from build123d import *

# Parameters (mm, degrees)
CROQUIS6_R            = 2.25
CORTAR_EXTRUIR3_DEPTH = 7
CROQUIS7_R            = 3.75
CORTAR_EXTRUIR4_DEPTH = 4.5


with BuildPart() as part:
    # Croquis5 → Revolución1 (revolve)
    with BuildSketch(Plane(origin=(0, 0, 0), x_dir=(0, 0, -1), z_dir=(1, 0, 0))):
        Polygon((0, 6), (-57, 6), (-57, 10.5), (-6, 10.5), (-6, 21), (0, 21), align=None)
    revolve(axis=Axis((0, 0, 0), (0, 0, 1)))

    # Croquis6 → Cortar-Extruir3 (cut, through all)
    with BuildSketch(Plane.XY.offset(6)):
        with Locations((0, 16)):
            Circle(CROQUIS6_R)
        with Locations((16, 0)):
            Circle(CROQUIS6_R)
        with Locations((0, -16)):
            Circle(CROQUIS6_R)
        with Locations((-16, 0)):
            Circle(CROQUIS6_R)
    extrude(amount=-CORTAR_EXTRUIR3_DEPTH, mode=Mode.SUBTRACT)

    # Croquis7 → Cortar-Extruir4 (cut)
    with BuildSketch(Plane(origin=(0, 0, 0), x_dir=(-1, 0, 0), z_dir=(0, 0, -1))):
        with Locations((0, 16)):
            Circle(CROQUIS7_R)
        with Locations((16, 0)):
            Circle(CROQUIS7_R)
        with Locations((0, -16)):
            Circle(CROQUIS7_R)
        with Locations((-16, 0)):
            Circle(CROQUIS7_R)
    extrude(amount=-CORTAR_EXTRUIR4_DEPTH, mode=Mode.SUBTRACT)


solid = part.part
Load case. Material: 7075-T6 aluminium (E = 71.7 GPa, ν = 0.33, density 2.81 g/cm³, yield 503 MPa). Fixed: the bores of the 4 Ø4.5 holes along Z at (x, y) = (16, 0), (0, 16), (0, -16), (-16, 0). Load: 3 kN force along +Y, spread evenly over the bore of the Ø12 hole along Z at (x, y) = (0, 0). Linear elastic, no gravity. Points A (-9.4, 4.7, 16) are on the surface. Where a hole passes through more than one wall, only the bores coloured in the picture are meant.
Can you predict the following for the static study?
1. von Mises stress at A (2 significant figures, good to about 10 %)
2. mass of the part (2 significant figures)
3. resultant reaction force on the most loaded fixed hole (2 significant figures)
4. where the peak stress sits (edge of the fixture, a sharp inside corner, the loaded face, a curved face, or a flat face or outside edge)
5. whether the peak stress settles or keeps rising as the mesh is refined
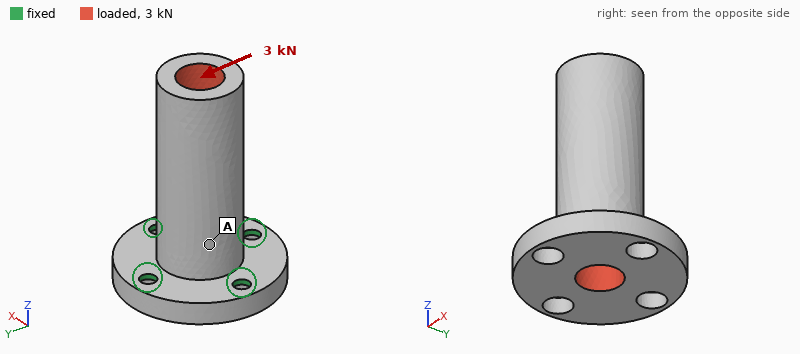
30 MPa
52 g
2.2 kN
edge of the fixture
keeps rising
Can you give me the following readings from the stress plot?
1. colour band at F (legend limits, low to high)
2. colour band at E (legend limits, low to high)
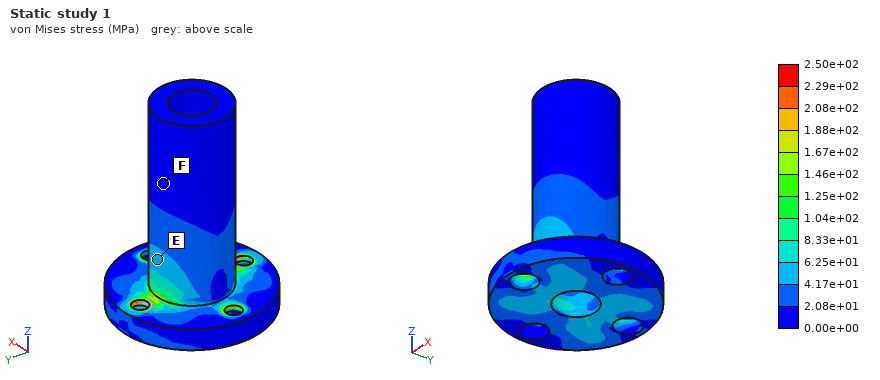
0.00e+00 to 2.08e+01 MPa
4.17e+01 to 6.25e+01 MPa
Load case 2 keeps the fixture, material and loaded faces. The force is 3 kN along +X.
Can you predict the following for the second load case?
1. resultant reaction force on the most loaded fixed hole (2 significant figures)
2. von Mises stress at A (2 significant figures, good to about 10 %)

2.2 kN
46 MPa
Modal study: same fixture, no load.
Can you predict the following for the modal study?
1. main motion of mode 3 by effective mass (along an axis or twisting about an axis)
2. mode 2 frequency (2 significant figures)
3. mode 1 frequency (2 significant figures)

along Z
3700 Hz
3700 Hz
